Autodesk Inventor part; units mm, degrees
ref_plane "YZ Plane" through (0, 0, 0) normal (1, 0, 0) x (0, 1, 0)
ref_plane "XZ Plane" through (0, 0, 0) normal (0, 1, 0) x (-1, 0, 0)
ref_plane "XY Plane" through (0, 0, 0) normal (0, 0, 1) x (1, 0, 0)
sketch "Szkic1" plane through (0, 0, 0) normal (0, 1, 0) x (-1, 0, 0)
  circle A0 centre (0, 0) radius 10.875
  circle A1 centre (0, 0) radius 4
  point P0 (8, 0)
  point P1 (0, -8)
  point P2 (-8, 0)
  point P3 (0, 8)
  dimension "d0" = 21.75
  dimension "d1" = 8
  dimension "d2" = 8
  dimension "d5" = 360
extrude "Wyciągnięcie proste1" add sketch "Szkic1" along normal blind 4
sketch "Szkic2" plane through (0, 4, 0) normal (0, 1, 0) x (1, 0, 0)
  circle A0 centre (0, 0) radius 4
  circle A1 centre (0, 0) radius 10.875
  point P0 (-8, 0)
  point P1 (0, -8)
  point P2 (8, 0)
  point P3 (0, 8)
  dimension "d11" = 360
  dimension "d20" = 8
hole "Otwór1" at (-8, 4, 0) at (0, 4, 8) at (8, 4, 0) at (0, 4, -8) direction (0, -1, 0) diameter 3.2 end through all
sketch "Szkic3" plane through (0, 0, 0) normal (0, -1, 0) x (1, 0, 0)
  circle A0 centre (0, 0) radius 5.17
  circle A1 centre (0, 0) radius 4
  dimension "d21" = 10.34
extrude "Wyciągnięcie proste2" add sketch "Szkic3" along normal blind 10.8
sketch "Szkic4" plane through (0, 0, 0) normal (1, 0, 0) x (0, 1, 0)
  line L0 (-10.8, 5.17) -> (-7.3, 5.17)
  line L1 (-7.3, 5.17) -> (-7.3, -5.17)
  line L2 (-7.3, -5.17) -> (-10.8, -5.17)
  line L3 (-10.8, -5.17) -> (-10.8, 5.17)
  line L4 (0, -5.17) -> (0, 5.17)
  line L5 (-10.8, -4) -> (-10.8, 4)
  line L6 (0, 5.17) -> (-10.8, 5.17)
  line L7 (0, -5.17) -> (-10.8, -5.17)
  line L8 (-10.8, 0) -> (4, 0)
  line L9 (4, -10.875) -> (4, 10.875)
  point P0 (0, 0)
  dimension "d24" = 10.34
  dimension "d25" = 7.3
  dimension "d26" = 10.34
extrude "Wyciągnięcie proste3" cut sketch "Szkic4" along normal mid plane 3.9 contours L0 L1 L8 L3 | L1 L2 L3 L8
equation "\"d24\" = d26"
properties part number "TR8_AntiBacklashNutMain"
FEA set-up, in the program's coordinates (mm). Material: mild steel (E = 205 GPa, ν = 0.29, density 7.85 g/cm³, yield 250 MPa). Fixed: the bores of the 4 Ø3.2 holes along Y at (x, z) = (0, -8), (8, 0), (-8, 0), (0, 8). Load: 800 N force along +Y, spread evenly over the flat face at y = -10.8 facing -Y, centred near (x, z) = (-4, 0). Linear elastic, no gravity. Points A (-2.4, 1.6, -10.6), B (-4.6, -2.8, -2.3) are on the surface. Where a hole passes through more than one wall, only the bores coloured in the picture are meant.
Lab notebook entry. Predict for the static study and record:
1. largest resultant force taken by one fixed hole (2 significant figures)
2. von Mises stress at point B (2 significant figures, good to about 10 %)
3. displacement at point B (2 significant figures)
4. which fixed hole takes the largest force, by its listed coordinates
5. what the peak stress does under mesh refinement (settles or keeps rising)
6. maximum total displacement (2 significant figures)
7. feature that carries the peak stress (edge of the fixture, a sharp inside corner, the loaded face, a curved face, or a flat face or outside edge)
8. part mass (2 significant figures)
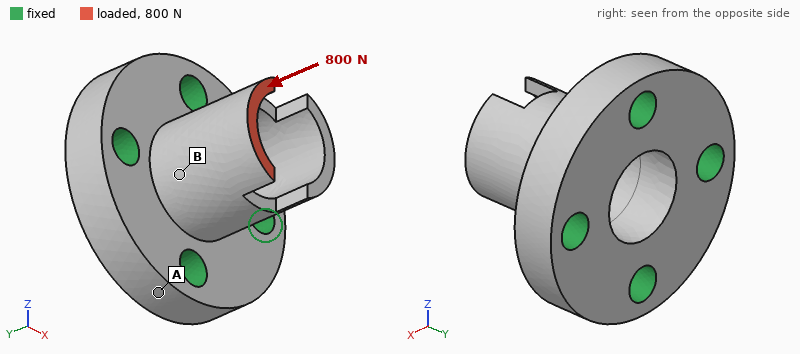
450 N
64 MPa
2.1 µm
(-8, 0)
keeps rising
6.9 µm
edge of the fixture
12 g
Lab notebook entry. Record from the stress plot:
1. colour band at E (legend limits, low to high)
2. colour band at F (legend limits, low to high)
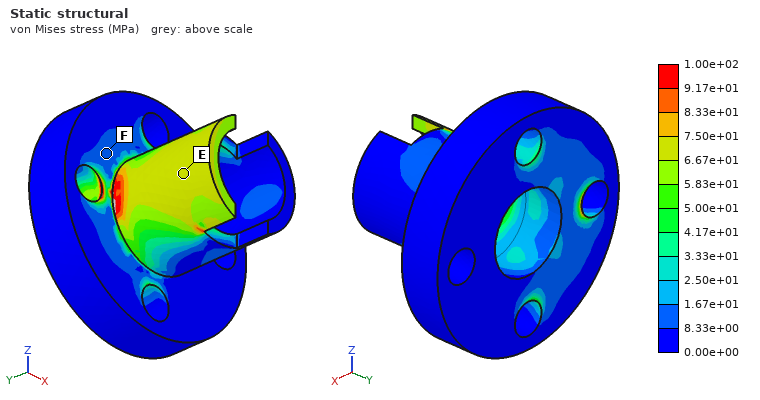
6.67e+01 to 7.50e+01 MPa
8.33e+00 to 1.67e+01 MPa
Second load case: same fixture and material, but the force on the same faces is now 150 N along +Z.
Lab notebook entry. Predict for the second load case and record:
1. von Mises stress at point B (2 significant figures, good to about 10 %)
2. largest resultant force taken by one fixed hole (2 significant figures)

29 MPa
150 N
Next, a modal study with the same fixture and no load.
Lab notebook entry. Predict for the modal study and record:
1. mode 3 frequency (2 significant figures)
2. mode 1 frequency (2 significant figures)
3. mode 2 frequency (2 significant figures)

37 kHz
34 kHz
37 kHz
